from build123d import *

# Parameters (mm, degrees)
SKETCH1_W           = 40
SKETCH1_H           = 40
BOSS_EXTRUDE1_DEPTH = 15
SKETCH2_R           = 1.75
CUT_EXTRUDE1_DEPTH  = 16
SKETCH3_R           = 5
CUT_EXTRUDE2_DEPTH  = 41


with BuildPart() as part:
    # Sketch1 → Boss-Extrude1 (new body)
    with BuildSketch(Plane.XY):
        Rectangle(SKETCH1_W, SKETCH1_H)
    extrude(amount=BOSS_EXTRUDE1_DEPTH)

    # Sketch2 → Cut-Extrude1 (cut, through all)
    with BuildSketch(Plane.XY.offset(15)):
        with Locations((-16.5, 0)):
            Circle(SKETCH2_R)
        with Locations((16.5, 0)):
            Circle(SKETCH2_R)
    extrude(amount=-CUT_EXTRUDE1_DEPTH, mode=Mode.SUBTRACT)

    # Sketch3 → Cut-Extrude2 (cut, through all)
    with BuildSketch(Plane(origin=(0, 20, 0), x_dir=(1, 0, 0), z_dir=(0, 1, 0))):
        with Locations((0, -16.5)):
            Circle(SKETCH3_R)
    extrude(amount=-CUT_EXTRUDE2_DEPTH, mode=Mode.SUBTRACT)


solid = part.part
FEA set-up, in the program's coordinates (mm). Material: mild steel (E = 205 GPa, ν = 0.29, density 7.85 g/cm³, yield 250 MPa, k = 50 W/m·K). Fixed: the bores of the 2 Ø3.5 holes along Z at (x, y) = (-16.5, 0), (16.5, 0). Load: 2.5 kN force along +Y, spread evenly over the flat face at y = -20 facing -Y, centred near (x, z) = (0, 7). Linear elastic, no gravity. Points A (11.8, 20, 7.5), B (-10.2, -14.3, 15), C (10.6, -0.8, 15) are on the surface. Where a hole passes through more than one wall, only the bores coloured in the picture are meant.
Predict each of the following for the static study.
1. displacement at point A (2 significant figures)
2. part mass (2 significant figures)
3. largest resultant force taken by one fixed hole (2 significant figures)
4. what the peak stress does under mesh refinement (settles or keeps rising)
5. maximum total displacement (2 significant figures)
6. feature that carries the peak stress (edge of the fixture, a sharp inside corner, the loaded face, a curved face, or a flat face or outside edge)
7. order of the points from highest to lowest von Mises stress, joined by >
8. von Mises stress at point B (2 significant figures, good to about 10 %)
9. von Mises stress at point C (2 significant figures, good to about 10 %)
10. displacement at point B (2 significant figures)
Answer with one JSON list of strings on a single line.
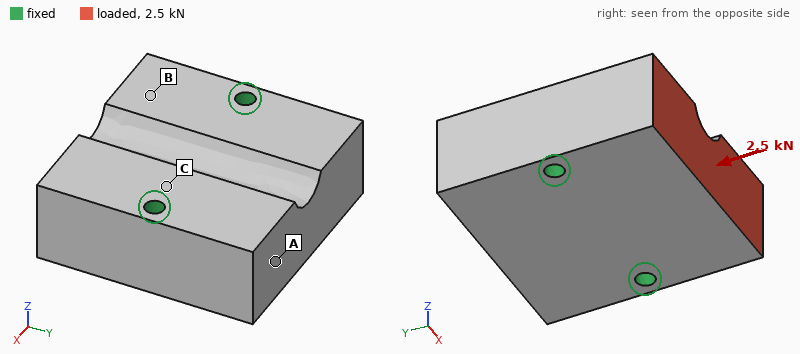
["0.19 µm", "180 g", "1.3 kN", "keeps rising", "0.69 µm", "edge of the fixture", "B > C > A", "4.2 MPa", "2.5 MPa", "0.44 µm"]
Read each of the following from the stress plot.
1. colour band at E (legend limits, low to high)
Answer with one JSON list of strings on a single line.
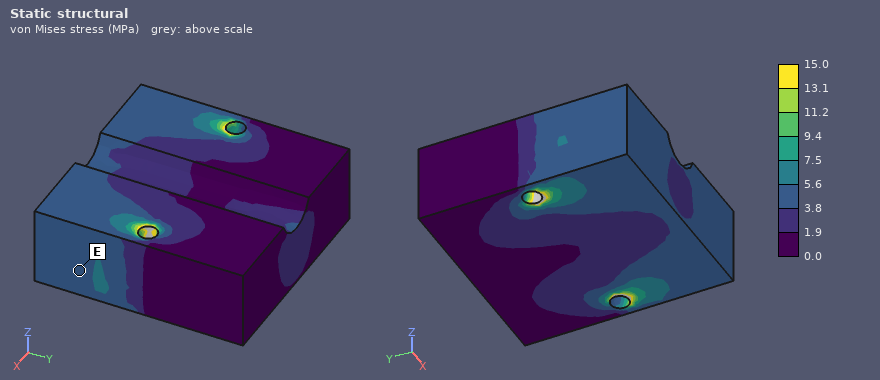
["3.8 to 5.6 MPa"]
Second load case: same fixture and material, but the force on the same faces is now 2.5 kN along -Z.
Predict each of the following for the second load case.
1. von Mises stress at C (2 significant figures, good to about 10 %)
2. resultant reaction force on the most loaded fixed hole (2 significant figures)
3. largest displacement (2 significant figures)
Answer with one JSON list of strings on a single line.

["19 MPa", "1.3 kN", "7.4 µm"]
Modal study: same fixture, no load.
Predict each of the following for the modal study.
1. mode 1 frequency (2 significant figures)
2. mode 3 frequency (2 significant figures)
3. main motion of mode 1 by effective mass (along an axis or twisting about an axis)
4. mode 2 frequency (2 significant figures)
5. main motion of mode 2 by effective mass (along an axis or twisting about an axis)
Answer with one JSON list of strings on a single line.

["16 kHz", "27 kHz", "twisting about X", "20 kHz", "along Z"]
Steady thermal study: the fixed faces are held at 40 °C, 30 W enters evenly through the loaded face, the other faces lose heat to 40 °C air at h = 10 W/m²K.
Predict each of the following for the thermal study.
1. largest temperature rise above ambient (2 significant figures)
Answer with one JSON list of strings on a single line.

["25 K"]
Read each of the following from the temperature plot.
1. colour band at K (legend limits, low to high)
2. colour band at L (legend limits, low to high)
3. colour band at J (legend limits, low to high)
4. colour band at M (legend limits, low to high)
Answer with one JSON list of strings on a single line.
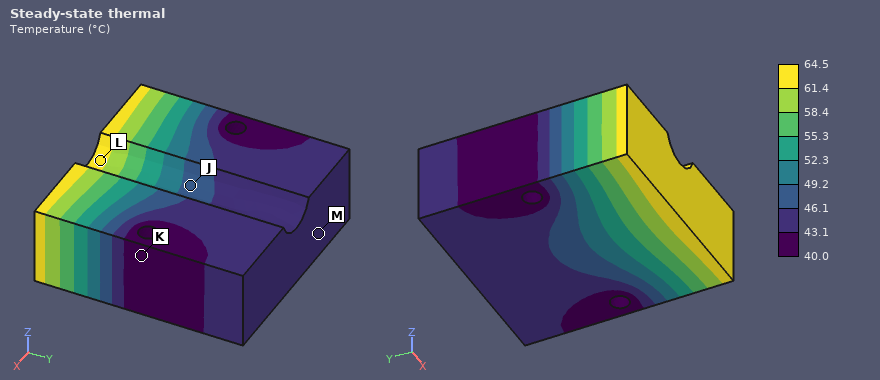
["40.0 to 43.1 °C", "61.4 to 64.5 °C", "46.1 to 49.2 °C", "43.1 to 46.1 °C"]
